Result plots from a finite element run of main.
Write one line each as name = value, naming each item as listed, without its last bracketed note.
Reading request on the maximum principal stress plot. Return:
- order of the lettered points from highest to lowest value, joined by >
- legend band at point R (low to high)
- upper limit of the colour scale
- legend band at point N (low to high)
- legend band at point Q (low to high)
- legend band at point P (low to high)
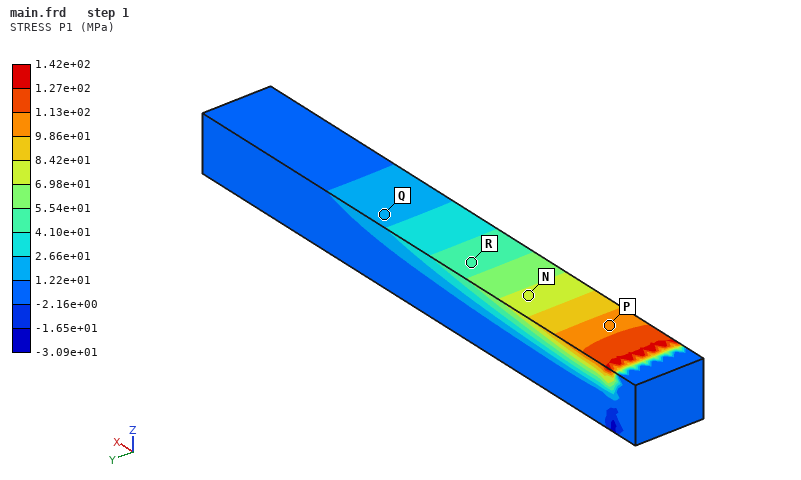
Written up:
order of the lettered points from highest to lowest value, joined by > = P > N > R > Q
legend band at point R = 4.10e+01 to 5.54e+01 MPa
upper limit of the colour scale = 1.42e+02 MPa
legend band at point N = 6.98e+01 to 8.42e+01 MPa
legend band at point Q = 1.22e+01 to 2.66e+01 MPa
legend band at point P = 9.86e+01 to 1.13e+02 MPa
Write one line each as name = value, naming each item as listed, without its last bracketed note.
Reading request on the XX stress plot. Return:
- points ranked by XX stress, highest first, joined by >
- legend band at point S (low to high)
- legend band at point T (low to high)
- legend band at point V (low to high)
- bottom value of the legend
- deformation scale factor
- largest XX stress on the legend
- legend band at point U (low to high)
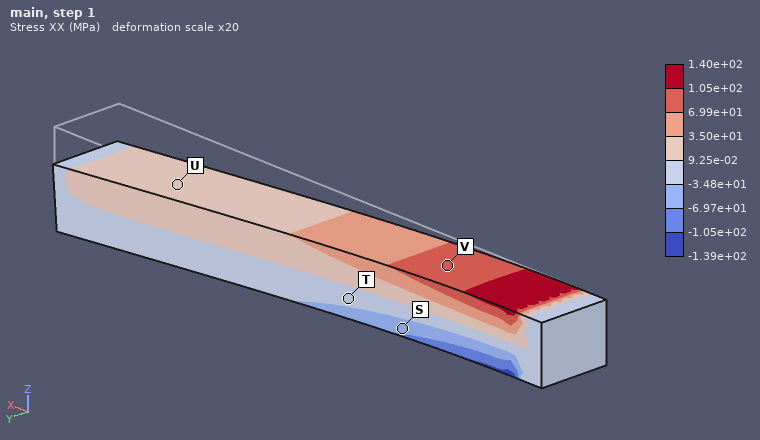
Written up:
points ranked by XX stress, highest first, joined by > = V > U > T > S
legend band at point S = -6.97e+01 to -3.48e+01 MPa
legend band at point T = -3.48e+01 to 9.25e-02 MPa
legend band at point V = 6.99e+01 to 1.05e+02 MPa
bottom value of the legend = -1.39e+02 MPa
deformation scale factor = 20
largest XX stress on the legend = 1.40e+02 MPa
legend band at point U = 9.25e-02 to 3.50e+01 MPa
